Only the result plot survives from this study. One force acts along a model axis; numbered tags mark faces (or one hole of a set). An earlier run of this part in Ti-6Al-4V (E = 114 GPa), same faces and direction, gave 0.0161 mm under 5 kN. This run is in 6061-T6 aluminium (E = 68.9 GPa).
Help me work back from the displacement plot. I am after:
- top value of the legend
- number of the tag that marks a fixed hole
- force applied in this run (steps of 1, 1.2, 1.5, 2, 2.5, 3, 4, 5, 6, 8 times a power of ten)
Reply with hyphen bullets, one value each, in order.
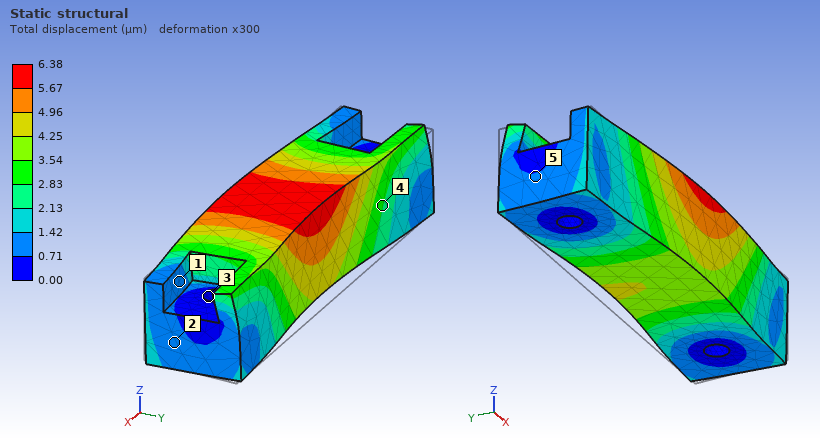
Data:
- 6.38 µm
- 3
- 1.2 kN
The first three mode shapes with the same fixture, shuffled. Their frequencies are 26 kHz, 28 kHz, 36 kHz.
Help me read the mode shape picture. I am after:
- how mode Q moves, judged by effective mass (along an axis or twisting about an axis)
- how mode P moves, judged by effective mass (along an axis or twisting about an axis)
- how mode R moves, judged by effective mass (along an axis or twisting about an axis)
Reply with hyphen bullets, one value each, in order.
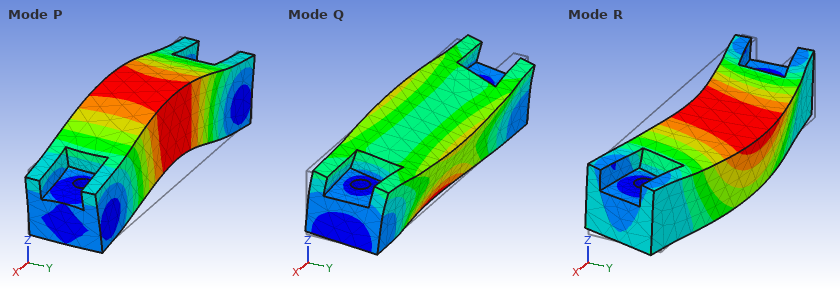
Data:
- twisting about X
- along Z
- along Y
